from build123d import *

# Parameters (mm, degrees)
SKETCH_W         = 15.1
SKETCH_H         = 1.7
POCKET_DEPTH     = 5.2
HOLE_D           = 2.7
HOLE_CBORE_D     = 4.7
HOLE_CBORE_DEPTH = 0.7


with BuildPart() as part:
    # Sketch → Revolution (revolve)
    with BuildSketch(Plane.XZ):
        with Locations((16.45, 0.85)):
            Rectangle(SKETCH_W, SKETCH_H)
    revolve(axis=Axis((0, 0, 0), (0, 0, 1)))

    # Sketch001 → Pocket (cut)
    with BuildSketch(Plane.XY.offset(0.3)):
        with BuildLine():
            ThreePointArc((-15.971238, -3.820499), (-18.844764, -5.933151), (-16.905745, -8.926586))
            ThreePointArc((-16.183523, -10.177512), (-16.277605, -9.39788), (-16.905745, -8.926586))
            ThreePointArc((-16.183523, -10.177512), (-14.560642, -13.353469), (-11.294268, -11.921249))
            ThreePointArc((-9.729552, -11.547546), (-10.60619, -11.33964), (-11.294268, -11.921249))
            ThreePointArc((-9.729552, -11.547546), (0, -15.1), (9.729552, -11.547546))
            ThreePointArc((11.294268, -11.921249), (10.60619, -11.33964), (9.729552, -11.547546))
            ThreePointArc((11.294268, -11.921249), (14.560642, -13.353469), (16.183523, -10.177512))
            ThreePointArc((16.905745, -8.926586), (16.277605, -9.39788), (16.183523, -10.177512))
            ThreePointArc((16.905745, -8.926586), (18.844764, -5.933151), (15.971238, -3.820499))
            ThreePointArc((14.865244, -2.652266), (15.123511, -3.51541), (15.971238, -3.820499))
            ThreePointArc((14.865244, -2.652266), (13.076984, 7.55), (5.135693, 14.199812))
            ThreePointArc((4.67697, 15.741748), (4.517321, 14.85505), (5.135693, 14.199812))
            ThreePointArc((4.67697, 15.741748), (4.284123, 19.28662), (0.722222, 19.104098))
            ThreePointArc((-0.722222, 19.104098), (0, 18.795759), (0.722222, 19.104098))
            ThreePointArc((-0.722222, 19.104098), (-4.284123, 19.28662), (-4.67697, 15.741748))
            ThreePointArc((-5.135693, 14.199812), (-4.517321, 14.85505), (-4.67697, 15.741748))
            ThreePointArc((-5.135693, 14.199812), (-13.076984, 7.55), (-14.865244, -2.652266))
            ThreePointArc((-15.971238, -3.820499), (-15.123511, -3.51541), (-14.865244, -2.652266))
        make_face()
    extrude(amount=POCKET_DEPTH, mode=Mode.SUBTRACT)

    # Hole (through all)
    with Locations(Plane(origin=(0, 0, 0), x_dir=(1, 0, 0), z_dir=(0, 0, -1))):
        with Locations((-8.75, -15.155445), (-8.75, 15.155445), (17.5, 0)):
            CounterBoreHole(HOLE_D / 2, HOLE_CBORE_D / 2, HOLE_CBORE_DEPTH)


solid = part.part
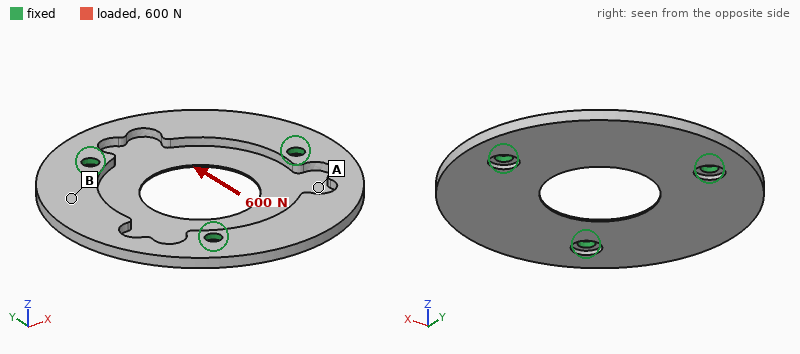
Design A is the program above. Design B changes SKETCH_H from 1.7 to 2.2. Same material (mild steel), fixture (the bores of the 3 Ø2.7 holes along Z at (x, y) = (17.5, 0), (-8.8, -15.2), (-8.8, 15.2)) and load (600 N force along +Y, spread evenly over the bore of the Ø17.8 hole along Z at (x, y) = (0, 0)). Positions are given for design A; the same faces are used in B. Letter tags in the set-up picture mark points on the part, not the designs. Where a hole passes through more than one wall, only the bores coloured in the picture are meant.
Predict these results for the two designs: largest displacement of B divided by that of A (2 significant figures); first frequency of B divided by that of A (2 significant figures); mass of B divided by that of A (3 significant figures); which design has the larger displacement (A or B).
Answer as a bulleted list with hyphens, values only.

- 0.62
- 1.2
- 1.35
- A
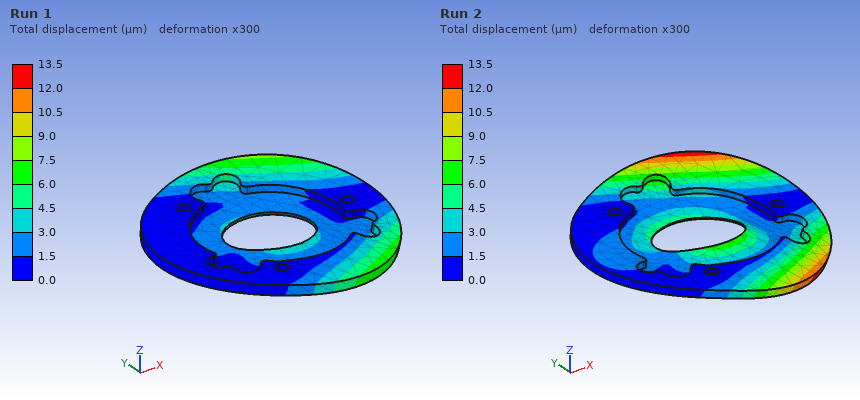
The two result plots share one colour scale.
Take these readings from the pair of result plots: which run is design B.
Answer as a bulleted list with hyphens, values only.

- Run 1
